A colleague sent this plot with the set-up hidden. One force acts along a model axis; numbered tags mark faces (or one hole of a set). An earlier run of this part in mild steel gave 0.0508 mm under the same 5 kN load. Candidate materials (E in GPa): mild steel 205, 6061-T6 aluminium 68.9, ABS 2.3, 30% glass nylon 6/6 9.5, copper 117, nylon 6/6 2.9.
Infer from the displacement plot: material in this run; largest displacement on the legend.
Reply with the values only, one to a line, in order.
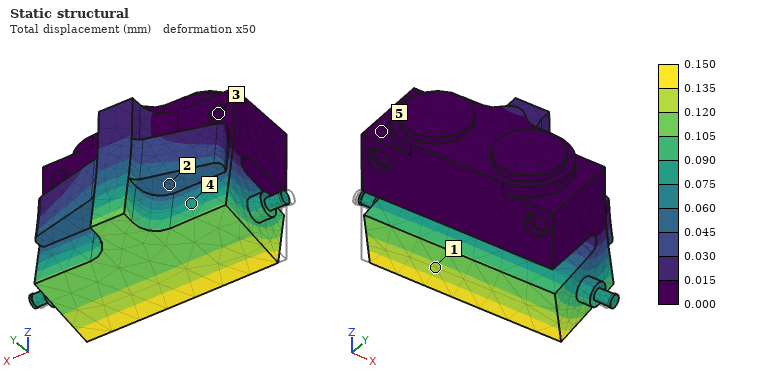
6061-T6 aluminium
0.150 mm
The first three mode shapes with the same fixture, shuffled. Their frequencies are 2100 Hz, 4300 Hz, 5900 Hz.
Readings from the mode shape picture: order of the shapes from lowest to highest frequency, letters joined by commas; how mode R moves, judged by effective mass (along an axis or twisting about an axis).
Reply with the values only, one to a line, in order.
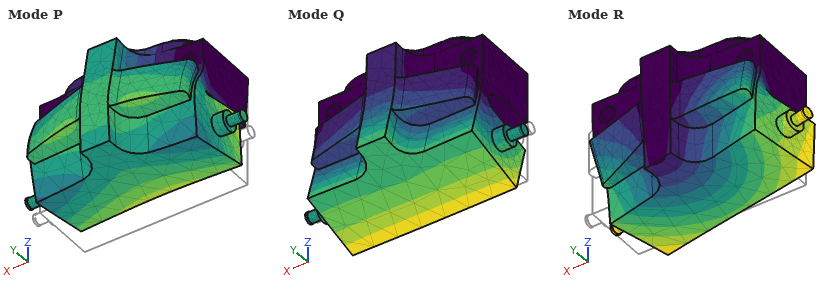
Q, R, P
along X
